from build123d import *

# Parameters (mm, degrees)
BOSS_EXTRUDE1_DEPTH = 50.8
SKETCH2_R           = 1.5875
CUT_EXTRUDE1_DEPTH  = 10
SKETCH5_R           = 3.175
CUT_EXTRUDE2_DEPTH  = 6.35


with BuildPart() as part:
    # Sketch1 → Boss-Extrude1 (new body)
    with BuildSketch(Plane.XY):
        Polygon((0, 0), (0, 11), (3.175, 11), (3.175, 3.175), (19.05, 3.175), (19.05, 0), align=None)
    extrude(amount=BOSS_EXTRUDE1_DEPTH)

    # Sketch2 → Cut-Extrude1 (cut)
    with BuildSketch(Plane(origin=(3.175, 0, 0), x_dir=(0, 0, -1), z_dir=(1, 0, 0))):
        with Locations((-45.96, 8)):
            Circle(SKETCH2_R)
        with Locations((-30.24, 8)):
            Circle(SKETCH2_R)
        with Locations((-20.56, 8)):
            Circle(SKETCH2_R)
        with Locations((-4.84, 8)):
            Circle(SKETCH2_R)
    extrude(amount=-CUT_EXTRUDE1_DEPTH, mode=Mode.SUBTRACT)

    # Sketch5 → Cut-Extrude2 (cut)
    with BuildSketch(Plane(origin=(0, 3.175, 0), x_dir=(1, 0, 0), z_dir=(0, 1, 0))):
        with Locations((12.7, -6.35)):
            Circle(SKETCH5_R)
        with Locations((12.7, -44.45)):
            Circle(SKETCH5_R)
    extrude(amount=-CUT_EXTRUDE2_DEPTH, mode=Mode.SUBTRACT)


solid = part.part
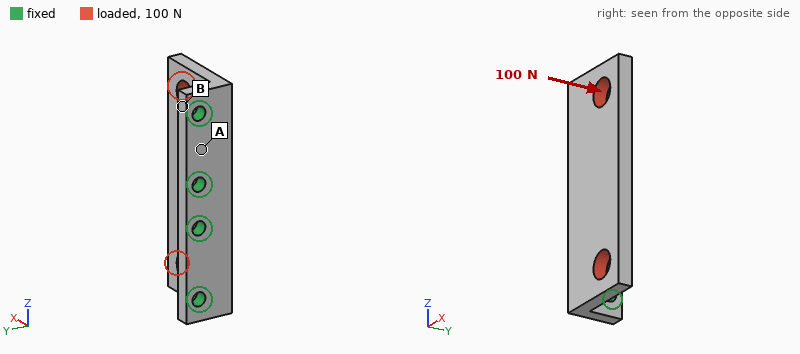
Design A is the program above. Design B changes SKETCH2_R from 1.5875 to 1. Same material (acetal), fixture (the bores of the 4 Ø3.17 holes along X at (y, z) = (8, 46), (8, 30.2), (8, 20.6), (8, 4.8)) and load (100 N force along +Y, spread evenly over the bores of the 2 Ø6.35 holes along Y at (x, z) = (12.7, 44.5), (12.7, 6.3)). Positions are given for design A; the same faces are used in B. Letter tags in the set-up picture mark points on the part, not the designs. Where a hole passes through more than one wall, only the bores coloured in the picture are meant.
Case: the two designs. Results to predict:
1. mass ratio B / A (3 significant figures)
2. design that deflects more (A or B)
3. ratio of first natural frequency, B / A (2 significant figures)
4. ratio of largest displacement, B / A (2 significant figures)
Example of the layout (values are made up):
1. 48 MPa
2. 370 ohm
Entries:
1. 1.02
2. B
3. 0.93
4. 1.1
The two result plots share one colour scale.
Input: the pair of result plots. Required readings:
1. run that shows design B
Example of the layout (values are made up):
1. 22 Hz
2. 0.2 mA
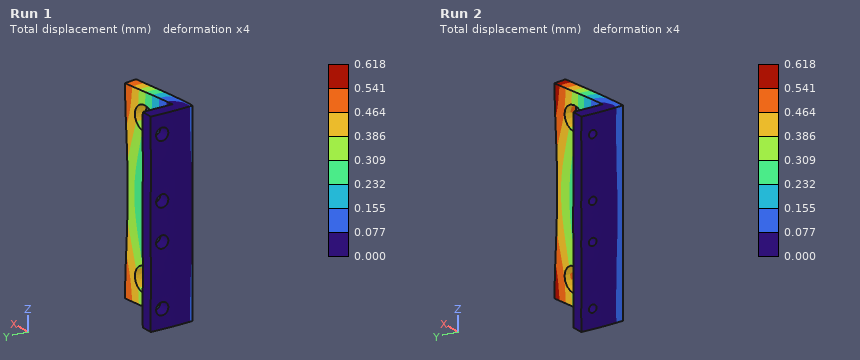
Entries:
1. Run 2
